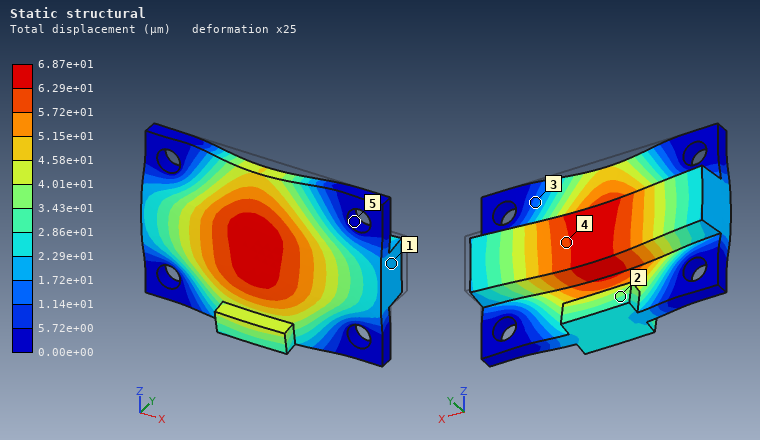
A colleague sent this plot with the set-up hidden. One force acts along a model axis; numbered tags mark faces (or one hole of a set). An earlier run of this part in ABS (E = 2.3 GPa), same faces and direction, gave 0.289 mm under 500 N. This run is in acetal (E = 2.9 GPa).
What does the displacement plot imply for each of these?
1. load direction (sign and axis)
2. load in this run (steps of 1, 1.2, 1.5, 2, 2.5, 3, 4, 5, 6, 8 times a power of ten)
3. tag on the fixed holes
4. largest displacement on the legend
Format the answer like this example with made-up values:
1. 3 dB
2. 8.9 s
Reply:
1. -Y
2. 150 N
3. 5
4. 6.87e+01 µm
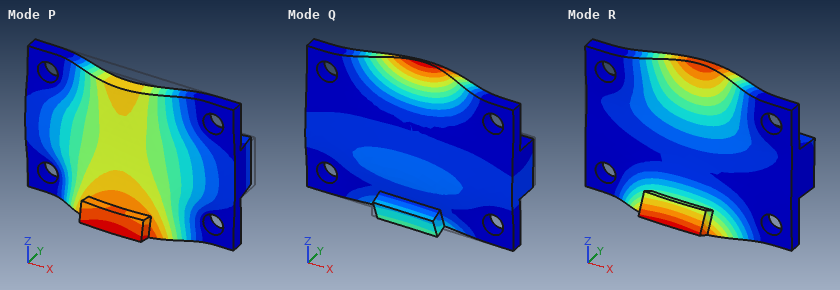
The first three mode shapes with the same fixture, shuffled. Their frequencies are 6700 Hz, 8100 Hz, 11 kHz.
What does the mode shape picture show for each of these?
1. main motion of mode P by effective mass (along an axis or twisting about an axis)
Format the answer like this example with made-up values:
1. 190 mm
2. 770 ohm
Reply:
1. along Y
